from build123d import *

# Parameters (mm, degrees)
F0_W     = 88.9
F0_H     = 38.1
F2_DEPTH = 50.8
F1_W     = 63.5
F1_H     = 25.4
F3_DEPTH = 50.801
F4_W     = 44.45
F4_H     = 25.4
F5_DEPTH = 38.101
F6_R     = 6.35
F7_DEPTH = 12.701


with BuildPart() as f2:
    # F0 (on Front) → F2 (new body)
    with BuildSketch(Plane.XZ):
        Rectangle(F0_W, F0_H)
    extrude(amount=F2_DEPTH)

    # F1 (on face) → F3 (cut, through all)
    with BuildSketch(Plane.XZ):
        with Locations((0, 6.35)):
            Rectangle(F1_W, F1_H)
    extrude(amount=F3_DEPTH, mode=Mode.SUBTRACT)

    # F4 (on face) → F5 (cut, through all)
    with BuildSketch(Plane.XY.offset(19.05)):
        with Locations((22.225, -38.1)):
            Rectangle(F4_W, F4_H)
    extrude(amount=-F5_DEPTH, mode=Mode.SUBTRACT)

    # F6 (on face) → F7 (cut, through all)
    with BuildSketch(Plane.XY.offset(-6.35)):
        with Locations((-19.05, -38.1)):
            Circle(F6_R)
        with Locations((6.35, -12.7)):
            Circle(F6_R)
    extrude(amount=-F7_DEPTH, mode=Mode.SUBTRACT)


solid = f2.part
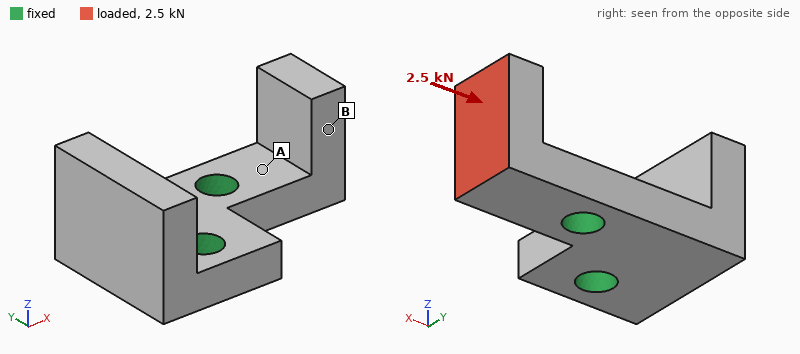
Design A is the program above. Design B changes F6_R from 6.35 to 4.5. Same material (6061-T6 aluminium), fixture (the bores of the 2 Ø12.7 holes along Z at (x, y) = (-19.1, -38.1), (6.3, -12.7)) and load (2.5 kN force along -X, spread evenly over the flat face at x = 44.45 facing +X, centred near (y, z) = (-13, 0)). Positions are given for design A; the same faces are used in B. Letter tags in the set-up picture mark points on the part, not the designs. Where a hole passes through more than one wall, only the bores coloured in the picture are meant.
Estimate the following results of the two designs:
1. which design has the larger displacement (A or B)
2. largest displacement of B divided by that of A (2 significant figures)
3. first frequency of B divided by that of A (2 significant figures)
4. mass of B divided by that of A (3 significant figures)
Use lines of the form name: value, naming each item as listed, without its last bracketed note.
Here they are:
which design has the larger displacement: B
largest displacement of B divided by that of A: 1.1
first frequency of B divided by that of A: 0.92
mass of B divided by that of A: 1.02
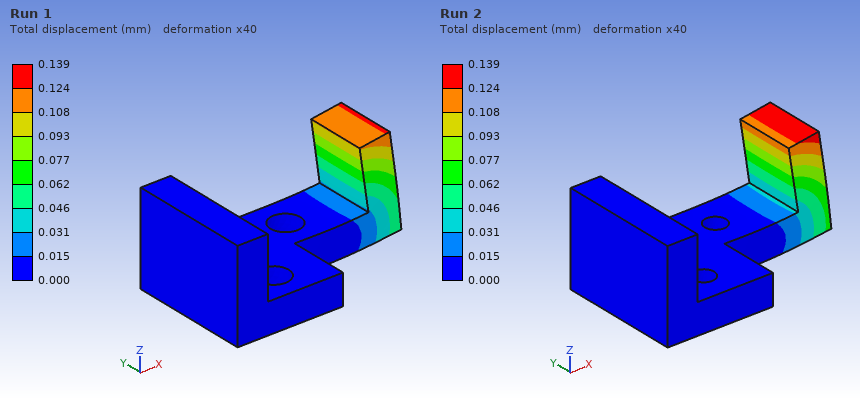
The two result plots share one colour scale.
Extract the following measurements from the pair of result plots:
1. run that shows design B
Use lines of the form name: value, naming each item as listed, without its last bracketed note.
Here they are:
run that shows design B: Run 2
